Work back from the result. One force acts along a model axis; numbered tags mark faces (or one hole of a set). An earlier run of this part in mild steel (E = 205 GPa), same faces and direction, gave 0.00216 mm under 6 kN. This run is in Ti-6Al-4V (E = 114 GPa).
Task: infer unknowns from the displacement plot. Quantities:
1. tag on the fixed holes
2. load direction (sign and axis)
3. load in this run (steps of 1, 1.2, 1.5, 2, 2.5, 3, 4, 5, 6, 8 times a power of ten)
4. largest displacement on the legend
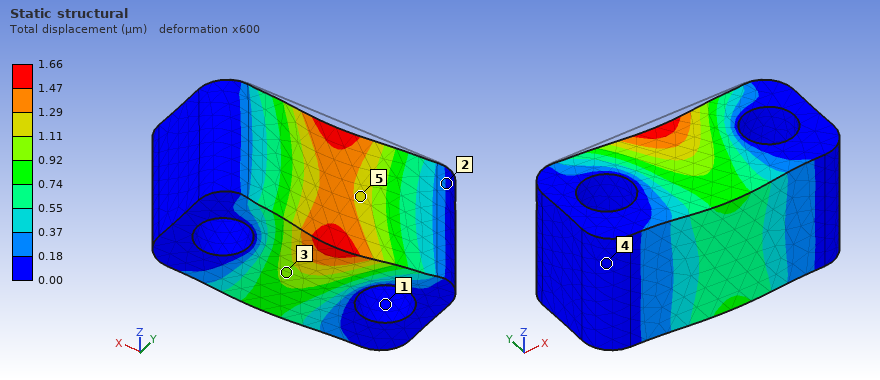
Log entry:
1
-Y
2.5 kN
1.66 µm
